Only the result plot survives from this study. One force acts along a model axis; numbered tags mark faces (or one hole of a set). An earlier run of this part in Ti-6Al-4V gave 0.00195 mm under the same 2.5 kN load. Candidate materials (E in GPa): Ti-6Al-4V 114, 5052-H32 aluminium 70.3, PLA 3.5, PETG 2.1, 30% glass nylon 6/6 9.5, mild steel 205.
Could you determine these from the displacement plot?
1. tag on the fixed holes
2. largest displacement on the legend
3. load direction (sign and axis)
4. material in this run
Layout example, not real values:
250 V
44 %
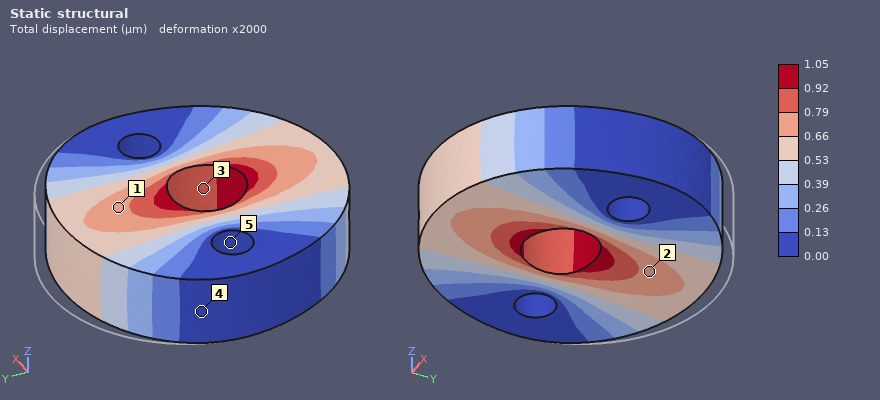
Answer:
5
1.05 µm
-Y
mild steel
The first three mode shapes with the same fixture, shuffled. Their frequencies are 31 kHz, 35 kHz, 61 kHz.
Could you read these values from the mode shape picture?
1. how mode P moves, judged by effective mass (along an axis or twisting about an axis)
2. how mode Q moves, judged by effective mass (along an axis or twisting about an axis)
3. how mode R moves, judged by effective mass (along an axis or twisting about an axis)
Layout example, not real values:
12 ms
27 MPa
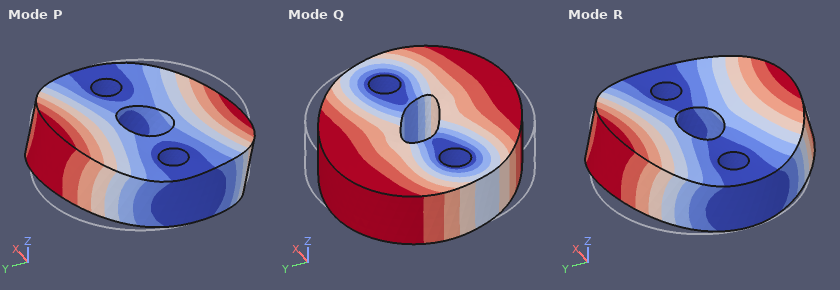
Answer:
twisting about X
twisting about Z
along Z
